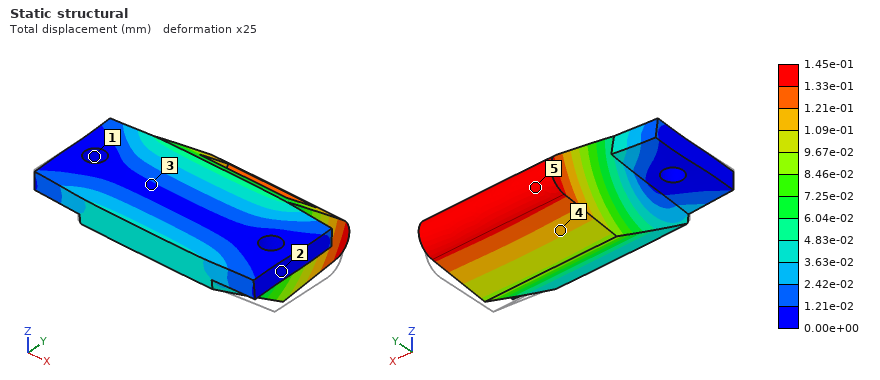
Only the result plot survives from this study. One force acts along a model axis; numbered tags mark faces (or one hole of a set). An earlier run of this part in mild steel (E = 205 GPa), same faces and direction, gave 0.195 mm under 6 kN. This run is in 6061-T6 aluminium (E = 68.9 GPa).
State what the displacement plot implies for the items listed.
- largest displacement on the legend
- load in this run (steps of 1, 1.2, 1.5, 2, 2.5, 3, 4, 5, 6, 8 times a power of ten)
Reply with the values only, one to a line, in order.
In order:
1.45e-01 mm
1.5 kN
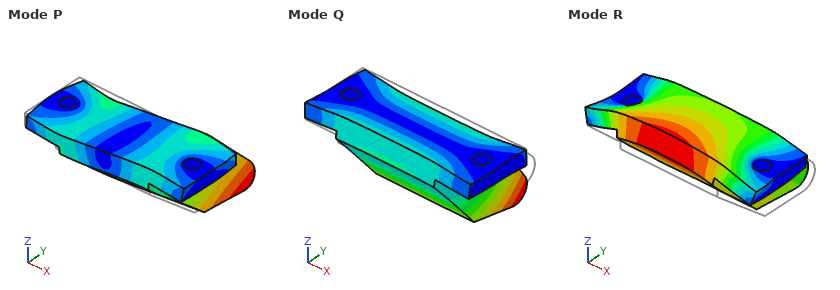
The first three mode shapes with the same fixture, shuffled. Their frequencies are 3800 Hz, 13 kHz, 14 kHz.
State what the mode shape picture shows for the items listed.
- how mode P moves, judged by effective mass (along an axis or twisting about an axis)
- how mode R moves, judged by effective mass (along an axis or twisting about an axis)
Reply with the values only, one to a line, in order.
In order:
along X
along Z
